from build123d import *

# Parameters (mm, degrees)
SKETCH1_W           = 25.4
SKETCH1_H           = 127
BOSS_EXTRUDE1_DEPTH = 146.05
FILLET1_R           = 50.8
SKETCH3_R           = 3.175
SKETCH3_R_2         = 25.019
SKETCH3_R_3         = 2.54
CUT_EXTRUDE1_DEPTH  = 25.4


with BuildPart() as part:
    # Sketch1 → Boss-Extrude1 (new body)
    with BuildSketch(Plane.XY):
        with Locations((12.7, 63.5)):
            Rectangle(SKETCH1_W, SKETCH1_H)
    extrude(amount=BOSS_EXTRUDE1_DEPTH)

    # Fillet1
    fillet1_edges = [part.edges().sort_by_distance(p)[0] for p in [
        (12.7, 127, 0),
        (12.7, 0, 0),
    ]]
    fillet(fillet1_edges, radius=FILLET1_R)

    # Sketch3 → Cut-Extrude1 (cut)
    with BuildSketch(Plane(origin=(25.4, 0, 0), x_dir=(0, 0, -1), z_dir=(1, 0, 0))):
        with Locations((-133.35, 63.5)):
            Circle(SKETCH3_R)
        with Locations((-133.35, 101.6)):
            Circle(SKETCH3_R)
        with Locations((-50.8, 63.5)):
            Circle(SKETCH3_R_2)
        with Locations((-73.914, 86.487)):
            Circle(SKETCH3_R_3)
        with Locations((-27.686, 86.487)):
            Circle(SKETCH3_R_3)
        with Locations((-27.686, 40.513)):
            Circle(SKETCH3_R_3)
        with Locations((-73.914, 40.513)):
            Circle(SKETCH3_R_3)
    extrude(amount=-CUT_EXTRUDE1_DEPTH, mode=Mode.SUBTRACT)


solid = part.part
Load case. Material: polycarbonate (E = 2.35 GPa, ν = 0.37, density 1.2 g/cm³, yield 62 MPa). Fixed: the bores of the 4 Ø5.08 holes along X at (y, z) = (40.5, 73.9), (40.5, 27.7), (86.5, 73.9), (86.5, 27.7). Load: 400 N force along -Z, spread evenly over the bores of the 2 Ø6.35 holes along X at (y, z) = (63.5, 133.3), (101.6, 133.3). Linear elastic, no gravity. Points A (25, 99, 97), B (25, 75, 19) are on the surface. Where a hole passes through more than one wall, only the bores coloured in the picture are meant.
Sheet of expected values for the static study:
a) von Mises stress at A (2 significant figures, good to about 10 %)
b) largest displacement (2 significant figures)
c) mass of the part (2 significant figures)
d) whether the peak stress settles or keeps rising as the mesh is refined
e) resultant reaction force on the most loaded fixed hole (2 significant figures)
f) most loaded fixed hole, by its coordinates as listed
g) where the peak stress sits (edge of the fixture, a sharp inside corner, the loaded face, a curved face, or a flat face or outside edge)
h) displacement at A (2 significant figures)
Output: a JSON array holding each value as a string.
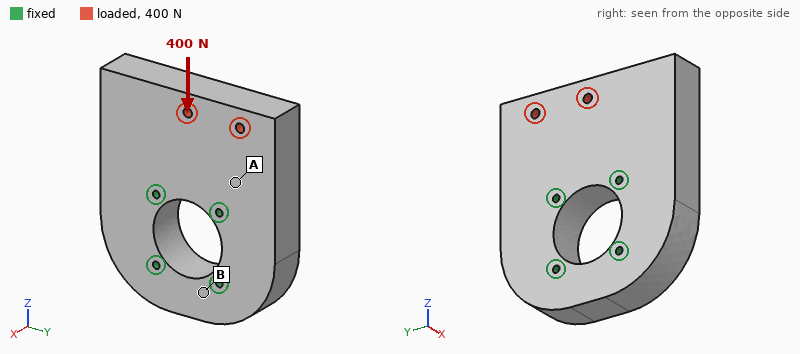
["0.23 MPa", "10 µm", "470 g", "keeps rising", "260 N", "(86.5, 73.9)", "edge of the fixture", "4.9 µm"]
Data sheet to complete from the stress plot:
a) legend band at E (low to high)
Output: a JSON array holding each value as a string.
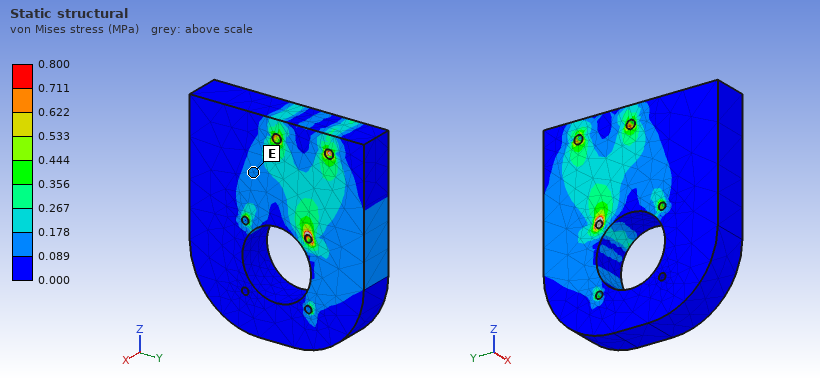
["0.089 to 0.178 MPa"]
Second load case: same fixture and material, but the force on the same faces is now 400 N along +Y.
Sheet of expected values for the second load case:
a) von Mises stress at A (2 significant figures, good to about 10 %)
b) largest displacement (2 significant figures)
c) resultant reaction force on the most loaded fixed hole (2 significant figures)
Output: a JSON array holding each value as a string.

["0.19 MPa", "31 µm", "360 N"]
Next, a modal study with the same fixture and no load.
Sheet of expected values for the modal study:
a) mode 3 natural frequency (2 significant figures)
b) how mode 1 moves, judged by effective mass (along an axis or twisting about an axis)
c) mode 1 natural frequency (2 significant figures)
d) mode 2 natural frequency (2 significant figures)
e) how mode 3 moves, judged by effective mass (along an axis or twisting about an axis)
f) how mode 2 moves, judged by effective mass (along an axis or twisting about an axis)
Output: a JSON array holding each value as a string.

["1600 Hz", "along X", "780 Hz", "1100 Hz", "along Y", "twisting about Z"]
